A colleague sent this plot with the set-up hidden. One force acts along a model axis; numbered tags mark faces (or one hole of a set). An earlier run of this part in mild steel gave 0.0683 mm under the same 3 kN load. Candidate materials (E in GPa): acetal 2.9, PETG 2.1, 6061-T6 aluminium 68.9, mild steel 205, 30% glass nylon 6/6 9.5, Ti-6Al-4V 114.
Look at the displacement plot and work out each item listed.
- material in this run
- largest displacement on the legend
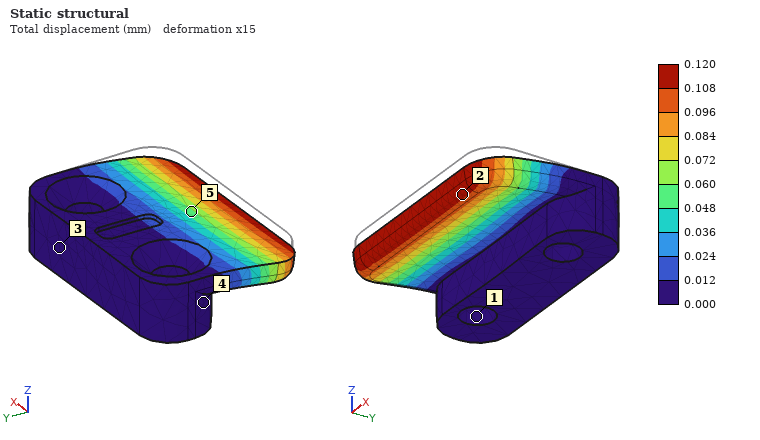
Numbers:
Ti-6Al-4V
0.120 mm
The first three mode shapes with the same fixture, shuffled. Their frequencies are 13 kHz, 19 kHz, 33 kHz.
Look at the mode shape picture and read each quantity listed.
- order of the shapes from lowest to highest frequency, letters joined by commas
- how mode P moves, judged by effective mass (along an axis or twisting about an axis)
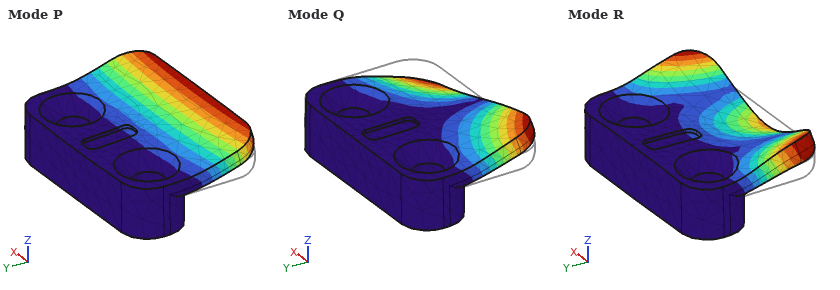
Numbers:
P, Q, R
along Z
